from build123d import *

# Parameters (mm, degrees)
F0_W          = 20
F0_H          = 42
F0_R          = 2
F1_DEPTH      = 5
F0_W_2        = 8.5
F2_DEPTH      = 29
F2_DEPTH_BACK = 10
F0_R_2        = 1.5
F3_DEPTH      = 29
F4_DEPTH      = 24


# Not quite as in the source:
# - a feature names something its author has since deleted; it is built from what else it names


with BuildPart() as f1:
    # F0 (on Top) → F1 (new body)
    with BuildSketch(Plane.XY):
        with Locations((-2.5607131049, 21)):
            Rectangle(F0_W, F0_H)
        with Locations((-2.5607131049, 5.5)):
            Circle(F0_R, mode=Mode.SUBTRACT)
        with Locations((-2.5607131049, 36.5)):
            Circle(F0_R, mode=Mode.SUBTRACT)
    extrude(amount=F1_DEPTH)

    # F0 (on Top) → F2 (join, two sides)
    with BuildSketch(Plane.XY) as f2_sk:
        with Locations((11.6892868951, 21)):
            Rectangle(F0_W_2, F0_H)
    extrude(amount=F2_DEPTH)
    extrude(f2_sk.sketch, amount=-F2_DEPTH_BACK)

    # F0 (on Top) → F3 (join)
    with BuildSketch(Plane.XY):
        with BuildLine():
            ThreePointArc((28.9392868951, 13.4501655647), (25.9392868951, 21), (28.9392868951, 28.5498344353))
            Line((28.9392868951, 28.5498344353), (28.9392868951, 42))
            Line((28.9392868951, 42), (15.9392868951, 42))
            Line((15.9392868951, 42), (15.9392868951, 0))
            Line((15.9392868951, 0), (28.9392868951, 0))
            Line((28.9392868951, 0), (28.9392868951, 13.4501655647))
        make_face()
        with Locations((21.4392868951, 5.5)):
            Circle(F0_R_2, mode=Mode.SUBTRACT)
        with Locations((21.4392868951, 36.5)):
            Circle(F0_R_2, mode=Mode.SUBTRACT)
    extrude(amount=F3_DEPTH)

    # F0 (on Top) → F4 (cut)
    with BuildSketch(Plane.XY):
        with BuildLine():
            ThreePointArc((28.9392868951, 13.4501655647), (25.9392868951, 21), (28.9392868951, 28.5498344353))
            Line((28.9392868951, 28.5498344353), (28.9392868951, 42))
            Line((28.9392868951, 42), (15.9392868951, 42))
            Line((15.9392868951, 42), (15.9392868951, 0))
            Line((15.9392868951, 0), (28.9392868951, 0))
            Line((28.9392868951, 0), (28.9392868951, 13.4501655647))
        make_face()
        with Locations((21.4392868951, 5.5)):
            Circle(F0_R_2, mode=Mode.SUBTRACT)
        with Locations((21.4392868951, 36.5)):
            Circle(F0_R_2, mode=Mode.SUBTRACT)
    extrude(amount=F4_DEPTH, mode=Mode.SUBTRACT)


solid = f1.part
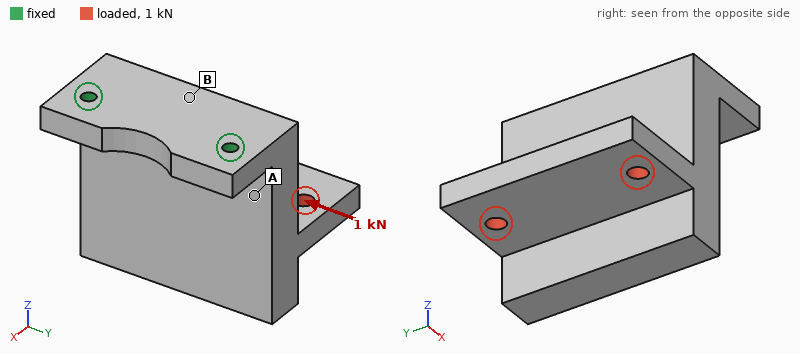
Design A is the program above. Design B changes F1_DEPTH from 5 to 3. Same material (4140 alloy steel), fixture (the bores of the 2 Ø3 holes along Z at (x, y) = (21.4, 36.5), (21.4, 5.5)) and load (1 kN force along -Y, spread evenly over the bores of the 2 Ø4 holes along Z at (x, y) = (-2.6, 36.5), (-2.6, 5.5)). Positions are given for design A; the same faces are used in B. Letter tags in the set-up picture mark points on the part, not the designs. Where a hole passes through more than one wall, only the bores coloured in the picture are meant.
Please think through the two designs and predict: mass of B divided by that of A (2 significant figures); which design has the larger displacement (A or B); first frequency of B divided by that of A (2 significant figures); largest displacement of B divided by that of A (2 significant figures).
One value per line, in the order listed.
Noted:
0.92
B
1.1
1.1
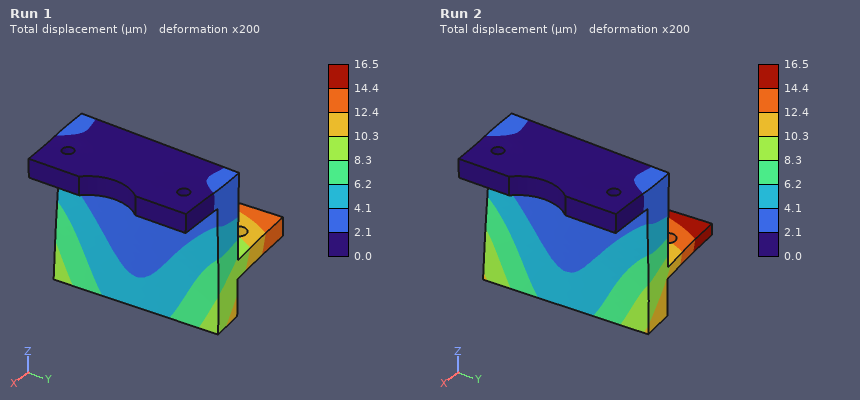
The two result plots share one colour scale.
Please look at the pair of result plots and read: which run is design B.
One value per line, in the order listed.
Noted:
Run 2
